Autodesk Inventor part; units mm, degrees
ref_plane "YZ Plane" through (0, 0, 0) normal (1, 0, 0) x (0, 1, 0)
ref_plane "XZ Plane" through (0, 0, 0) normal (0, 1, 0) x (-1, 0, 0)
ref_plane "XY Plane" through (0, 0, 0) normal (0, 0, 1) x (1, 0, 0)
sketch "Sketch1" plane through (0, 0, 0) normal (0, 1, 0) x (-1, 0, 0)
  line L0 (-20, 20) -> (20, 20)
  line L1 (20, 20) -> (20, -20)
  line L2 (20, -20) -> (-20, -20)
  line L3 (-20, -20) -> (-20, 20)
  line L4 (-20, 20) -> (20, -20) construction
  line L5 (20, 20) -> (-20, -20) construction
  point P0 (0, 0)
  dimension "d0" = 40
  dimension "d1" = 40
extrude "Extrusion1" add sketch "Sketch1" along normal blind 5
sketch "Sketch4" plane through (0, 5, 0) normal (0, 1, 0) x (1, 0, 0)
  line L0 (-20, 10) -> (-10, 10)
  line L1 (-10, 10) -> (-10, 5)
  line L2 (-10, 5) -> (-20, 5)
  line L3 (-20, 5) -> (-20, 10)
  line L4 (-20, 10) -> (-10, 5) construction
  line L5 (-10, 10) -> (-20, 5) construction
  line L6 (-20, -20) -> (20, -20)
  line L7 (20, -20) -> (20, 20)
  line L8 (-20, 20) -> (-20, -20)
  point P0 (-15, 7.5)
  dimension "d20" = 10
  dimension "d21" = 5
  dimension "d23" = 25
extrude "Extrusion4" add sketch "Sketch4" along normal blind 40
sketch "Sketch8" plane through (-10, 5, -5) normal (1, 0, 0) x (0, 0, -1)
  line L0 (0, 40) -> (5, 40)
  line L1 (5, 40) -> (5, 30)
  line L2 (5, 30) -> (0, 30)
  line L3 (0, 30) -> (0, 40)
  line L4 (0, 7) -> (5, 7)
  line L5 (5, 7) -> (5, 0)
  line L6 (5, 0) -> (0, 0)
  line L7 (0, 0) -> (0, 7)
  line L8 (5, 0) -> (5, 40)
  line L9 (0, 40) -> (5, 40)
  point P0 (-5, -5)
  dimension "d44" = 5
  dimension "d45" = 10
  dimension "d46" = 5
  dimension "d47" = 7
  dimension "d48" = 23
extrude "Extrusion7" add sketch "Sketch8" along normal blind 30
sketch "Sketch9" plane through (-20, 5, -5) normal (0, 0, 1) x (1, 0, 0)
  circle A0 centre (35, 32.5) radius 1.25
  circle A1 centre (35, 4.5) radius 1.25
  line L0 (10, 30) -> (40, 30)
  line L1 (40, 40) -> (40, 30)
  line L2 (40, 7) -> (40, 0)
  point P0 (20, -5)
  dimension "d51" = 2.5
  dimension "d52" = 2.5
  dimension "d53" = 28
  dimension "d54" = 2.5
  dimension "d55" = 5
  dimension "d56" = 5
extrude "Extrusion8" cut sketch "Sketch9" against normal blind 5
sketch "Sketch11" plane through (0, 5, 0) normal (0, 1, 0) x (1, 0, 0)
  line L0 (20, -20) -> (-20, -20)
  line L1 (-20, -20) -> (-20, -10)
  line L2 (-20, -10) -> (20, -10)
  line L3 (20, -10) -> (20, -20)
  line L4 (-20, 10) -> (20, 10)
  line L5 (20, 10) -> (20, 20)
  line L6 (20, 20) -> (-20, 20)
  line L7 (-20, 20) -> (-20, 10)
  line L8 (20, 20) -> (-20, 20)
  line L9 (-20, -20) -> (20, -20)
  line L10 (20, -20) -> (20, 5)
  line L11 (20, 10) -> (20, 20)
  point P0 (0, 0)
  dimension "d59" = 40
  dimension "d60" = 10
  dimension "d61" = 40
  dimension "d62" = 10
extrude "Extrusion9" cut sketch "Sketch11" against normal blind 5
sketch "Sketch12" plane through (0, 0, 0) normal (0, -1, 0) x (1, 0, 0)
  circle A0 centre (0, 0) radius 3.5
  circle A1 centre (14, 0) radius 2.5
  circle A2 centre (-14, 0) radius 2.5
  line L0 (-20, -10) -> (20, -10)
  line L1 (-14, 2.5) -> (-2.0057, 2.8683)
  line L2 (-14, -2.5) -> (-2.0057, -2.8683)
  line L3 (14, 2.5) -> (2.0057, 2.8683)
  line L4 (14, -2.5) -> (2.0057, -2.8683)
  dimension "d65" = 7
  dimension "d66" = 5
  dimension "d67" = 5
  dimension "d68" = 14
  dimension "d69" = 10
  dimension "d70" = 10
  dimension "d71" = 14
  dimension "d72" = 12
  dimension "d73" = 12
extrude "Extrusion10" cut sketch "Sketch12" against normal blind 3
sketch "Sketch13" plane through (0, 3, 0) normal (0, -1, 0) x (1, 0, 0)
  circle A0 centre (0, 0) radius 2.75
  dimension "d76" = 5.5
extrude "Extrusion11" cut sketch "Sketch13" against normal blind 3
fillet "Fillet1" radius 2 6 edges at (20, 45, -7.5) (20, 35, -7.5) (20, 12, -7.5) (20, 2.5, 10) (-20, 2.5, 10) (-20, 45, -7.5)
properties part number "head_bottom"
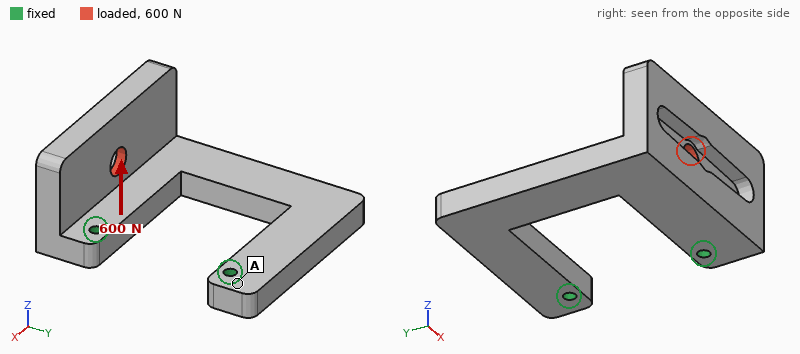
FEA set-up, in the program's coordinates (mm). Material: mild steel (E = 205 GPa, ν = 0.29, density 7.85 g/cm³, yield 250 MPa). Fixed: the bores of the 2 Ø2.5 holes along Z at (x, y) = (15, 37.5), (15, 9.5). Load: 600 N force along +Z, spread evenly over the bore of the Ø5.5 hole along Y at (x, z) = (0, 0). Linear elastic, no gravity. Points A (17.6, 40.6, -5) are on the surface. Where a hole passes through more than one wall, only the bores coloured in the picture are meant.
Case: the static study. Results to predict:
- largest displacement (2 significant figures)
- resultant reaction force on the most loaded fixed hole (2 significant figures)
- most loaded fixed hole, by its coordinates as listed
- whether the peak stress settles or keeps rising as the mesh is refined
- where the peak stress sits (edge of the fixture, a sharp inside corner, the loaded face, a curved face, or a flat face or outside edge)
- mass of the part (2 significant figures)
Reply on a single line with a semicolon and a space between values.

69 µm; 580 N; (15, 9.5); keeps rising; edge of the fixture; 62 g
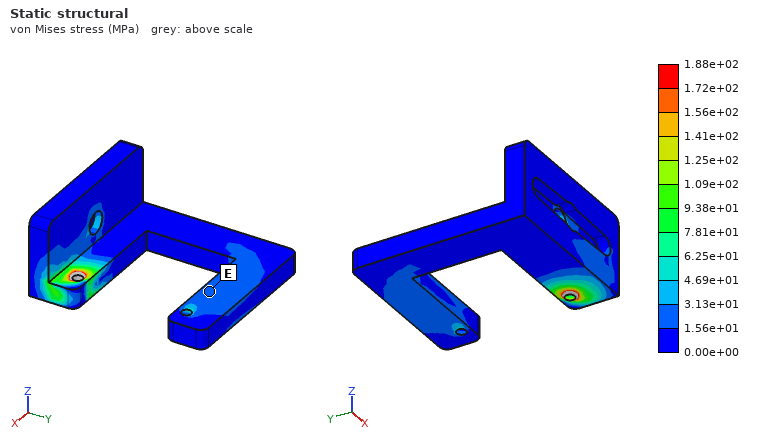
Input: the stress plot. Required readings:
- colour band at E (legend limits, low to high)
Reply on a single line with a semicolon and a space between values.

1.56e+01 to 3.13e+01 MPa
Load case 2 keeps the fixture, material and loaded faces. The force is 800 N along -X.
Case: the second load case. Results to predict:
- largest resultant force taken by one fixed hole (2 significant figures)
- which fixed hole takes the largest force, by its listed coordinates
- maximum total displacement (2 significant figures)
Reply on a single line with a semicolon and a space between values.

850 N; (15, 9.5); 46 µm
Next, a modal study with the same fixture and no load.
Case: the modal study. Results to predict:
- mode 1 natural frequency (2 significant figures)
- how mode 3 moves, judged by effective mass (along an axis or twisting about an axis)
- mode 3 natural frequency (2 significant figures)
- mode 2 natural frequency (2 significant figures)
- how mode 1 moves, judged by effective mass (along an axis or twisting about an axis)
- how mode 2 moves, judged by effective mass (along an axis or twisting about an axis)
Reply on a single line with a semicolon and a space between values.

2400 Hz; along Y; 4600 Hz; 3600 Hz; along Z; along Y
